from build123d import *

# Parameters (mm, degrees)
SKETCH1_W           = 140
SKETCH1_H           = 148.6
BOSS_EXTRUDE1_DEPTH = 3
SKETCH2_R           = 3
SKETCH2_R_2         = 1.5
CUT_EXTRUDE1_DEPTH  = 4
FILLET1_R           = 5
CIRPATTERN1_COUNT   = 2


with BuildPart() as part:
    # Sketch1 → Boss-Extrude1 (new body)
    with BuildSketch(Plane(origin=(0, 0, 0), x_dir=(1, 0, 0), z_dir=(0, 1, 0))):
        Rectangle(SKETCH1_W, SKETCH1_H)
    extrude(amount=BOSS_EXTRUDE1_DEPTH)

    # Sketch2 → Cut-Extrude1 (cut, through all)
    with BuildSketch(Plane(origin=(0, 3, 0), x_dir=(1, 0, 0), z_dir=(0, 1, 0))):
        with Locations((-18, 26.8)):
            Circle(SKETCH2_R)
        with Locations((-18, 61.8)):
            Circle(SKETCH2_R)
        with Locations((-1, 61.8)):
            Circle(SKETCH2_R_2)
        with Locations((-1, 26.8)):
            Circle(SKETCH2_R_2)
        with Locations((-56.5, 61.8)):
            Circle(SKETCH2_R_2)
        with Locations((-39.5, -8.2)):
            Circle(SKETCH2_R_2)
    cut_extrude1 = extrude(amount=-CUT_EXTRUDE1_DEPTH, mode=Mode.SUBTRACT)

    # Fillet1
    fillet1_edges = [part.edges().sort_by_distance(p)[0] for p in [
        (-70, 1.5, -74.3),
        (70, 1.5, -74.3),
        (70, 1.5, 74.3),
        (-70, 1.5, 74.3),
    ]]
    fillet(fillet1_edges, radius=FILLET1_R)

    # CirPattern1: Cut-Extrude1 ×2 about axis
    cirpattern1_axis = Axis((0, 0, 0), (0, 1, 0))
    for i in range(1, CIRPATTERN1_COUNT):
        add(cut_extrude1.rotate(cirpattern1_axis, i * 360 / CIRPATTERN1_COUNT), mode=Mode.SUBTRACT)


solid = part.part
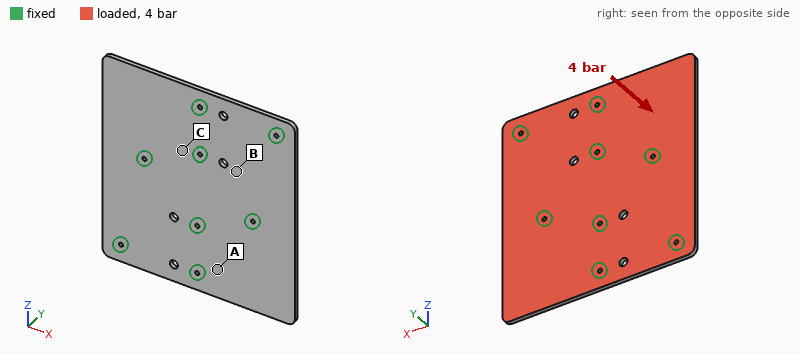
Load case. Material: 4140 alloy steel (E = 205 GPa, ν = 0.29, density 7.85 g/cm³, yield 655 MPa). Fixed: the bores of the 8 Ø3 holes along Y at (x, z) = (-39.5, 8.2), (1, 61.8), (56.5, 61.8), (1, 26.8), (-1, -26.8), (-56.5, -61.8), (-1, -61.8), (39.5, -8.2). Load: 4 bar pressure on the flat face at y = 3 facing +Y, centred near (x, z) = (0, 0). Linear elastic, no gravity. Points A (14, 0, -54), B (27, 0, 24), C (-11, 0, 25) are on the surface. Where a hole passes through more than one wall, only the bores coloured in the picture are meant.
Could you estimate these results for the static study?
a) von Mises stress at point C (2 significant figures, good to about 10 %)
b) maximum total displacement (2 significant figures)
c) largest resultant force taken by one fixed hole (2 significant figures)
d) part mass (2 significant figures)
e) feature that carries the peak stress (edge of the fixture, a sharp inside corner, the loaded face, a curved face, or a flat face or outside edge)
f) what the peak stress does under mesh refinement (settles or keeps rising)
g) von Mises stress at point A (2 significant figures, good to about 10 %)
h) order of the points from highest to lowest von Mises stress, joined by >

84 MPa
0.98 mm
1.9 kN
490 g
edge of the fixture
keeps rising
150 MPa
A > C > B
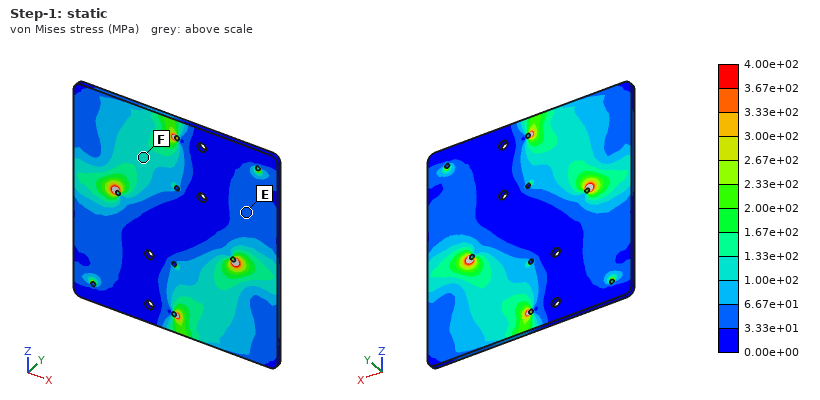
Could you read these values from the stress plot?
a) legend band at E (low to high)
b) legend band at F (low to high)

3.33e+01 to 6.67e+01 MPa
1.00e+02 to 1.33e+02 MPa
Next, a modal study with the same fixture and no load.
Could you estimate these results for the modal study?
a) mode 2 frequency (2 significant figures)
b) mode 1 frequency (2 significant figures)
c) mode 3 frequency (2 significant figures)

920 Hz
920 Hz
2300 Hz
